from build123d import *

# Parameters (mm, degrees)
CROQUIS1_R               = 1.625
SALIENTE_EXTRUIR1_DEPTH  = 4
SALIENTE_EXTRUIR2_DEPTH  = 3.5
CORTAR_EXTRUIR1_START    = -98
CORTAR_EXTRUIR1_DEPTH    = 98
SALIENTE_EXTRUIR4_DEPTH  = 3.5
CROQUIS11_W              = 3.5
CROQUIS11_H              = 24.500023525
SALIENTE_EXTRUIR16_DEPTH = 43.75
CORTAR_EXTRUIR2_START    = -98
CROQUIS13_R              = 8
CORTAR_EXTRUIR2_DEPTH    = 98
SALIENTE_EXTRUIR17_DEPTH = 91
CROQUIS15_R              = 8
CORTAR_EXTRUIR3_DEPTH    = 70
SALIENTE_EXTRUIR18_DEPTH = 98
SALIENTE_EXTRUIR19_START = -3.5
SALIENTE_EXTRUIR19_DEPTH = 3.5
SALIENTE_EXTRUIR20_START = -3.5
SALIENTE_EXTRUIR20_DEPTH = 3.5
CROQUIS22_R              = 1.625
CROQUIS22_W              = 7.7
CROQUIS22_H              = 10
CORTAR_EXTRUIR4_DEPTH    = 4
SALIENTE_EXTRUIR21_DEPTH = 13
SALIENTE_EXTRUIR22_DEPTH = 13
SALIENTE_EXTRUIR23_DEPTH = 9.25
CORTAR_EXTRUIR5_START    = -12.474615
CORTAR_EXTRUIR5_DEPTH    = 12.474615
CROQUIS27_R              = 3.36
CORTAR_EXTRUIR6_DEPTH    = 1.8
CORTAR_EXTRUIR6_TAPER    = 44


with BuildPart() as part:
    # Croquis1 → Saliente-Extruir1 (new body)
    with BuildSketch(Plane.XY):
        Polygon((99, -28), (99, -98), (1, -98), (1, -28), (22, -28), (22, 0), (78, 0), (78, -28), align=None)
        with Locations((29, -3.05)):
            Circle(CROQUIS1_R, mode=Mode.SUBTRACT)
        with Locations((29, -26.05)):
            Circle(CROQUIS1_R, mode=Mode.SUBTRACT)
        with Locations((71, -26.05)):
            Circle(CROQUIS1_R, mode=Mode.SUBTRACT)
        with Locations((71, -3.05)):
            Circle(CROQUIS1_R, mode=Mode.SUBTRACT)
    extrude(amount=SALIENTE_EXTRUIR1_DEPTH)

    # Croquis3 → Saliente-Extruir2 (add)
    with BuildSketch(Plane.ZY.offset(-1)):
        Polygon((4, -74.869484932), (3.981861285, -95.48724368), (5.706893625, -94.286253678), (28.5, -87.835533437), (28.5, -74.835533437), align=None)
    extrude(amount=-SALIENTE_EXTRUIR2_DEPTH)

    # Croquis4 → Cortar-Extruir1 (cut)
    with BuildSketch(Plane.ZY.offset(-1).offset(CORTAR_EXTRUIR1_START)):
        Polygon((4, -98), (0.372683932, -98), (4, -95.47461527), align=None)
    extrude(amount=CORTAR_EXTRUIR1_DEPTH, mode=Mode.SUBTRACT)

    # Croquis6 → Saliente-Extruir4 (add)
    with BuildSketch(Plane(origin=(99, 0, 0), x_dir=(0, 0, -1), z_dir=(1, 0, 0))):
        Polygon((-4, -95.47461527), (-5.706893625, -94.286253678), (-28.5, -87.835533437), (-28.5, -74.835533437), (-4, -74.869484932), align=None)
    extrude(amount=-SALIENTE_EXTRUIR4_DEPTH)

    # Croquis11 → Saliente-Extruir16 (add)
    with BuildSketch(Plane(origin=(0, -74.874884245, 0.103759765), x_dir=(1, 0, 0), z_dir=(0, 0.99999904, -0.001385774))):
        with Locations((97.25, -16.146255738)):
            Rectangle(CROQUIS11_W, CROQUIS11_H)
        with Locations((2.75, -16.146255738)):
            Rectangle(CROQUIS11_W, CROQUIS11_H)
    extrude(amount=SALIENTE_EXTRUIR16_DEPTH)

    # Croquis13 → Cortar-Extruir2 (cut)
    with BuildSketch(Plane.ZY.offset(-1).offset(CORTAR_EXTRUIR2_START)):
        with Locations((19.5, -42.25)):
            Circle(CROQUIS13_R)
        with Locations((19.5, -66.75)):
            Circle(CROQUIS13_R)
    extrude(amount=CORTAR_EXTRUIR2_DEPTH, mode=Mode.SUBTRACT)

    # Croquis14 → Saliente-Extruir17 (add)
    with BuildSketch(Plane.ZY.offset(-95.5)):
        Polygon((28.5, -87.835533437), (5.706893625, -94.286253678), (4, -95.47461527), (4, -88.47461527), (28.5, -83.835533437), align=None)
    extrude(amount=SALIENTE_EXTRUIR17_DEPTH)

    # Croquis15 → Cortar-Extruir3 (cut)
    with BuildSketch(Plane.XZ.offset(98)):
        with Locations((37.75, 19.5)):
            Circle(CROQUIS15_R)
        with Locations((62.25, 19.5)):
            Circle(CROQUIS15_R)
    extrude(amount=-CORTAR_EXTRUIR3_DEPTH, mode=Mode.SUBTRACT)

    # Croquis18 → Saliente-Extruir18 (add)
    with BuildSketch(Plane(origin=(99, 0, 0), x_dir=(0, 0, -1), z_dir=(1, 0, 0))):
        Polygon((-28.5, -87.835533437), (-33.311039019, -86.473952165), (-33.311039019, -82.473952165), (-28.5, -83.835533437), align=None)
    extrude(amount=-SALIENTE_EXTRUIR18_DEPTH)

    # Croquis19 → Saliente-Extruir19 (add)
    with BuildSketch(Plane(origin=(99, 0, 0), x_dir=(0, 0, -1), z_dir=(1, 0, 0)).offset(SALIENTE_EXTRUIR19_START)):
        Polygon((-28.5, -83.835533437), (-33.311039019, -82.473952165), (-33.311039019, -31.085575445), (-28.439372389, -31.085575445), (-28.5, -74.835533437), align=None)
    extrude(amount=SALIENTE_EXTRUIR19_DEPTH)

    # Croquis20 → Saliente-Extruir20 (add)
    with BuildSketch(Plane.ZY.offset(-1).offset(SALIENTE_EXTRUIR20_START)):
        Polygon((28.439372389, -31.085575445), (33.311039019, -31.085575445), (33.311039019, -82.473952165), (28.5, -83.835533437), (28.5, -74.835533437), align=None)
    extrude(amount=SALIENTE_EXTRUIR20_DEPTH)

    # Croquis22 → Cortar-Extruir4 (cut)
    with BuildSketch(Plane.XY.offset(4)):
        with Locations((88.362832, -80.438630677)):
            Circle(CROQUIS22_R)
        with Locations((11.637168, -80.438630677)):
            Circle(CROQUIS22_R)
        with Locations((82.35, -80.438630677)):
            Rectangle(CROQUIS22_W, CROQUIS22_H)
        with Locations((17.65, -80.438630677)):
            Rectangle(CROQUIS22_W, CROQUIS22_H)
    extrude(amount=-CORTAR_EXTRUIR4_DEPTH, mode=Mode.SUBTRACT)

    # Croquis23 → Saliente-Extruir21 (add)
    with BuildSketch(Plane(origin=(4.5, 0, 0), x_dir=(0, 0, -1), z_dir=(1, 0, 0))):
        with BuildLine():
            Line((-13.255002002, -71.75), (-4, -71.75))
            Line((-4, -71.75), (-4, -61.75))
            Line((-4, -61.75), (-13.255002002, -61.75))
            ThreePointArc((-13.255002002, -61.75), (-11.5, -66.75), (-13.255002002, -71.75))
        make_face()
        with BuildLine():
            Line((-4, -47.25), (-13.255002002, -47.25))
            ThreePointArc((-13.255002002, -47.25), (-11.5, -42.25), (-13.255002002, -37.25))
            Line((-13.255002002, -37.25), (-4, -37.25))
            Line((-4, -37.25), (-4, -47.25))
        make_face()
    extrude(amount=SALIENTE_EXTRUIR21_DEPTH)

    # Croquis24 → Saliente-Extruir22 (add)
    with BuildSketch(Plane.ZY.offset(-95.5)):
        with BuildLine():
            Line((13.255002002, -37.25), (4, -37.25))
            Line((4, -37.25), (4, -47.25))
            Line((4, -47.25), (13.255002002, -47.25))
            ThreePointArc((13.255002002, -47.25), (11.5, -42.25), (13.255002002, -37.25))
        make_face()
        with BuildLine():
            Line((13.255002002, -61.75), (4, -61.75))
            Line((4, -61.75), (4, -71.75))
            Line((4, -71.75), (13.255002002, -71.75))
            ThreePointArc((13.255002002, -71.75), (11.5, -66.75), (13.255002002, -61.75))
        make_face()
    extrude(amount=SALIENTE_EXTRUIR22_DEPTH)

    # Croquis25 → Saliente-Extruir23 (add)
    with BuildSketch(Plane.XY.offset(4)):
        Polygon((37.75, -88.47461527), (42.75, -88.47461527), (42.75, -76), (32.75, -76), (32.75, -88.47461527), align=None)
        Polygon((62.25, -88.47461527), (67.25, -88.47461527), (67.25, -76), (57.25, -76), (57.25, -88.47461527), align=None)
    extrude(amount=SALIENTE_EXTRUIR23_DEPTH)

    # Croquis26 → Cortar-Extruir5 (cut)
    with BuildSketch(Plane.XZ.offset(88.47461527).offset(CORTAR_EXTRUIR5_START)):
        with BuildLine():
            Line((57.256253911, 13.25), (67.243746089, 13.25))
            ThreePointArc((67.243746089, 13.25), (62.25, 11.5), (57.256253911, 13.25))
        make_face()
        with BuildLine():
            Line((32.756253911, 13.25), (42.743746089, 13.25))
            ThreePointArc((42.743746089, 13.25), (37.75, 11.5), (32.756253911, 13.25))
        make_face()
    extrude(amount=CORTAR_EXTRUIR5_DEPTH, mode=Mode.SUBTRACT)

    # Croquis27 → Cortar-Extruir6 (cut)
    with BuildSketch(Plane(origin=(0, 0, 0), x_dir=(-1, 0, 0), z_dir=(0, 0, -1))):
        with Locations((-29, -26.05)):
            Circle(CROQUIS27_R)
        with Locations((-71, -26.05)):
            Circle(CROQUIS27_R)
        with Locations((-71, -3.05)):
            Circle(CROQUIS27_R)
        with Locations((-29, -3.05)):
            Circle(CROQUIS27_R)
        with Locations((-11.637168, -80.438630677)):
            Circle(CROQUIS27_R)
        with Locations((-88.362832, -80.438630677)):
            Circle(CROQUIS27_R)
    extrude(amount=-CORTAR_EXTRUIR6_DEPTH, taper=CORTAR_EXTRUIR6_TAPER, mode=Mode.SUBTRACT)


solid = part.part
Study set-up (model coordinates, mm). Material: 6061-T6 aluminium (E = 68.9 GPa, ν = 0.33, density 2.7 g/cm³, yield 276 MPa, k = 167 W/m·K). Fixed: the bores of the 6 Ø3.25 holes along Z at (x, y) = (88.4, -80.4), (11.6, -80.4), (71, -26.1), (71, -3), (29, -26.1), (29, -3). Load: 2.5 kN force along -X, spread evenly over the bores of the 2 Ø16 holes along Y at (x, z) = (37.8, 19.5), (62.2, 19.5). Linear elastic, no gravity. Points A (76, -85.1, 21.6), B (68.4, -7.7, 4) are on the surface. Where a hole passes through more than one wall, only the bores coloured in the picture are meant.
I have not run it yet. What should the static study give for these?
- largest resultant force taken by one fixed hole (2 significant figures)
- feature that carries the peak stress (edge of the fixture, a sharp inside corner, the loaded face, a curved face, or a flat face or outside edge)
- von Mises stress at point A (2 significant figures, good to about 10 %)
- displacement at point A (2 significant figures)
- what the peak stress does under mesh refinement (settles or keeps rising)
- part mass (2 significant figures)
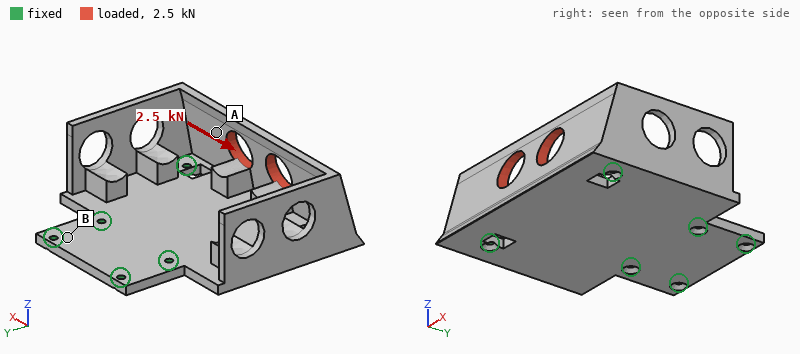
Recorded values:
1.2 kN
edge of the fixture
11 MPa
23 µm
keeps rising
160 g
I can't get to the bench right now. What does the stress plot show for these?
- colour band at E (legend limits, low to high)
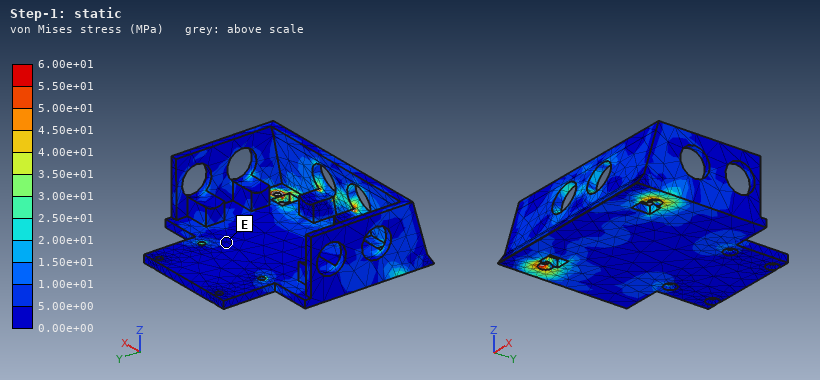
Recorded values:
0.00e+00 to 5.00e+00 MPa
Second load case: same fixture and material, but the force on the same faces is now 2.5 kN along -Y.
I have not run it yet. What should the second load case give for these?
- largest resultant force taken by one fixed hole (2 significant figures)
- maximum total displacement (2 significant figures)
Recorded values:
740 N
0.33 mm
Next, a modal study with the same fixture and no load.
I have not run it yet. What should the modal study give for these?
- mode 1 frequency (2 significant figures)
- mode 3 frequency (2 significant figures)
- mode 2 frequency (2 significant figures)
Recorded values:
2300 Hz
3800 Hz
2700 Hz
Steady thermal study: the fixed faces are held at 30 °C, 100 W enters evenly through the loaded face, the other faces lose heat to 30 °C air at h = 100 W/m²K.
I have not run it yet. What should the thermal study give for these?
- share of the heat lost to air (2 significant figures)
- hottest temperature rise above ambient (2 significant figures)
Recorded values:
48 %
67 K
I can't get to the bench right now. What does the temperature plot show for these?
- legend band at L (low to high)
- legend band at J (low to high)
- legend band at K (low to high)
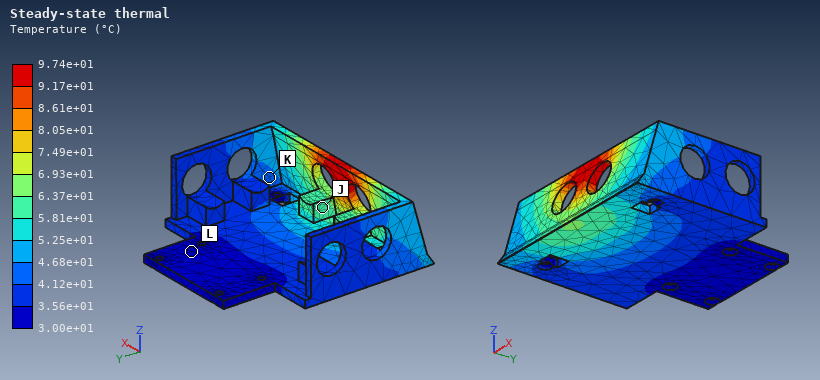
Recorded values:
3.00e+01 to 3.56e+01 °C
5.81e+01 to 6.37e+01 °C
4.12e+01 to 4.68e+01 °C
